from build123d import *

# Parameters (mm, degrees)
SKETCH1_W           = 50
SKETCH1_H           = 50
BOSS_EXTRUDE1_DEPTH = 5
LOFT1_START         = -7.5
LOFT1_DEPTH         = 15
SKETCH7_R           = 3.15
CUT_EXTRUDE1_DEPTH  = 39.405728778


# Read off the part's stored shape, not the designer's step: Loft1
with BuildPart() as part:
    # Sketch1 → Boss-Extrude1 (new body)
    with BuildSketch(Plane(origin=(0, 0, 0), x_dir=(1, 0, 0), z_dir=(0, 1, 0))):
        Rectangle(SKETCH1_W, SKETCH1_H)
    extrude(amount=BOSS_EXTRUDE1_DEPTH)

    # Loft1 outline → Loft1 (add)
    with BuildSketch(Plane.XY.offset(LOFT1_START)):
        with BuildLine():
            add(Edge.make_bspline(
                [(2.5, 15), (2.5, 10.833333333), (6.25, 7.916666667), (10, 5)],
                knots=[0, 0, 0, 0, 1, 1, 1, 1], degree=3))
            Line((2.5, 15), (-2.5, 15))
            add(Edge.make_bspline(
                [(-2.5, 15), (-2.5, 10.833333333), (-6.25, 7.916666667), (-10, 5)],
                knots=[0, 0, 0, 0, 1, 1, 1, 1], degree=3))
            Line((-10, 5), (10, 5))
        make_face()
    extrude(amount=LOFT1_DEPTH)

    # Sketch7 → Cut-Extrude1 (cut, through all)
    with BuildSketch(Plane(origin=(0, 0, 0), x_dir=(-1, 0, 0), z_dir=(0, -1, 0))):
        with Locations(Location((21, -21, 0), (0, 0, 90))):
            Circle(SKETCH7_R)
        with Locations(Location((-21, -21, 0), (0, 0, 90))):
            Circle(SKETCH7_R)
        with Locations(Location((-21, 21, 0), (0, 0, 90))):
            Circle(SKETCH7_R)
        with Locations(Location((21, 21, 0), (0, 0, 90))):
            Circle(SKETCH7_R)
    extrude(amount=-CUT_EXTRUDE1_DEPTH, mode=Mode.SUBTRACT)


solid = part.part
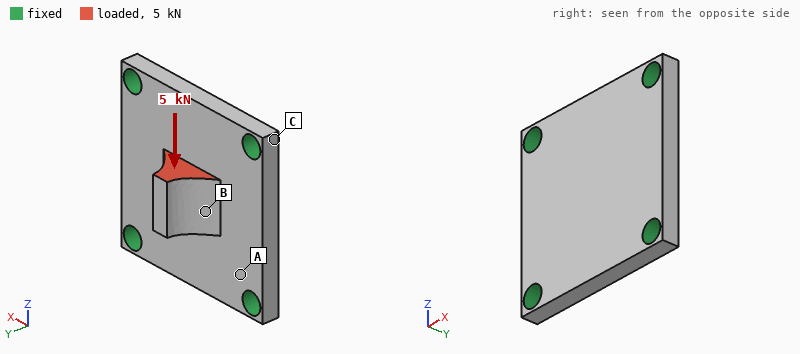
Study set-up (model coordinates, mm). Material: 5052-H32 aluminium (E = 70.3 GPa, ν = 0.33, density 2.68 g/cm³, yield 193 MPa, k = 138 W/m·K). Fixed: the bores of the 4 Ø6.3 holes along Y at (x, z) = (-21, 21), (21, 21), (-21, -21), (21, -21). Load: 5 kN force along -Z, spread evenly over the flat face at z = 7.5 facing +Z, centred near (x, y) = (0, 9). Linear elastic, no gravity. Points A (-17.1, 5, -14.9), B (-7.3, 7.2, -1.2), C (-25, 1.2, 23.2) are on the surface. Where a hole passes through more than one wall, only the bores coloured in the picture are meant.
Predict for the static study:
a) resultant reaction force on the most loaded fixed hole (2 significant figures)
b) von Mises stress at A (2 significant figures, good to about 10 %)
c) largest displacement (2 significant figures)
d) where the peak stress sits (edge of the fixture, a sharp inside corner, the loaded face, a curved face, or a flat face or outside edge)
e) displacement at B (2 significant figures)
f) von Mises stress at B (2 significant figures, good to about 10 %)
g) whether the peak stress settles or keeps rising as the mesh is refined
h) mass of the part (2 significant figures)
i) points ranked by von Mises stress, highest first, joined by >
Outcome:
1.5 kN
28 MPa
50 µm
edge of the fixture
17 µm
48 MPa
keeps rising
36 g
B > A > C
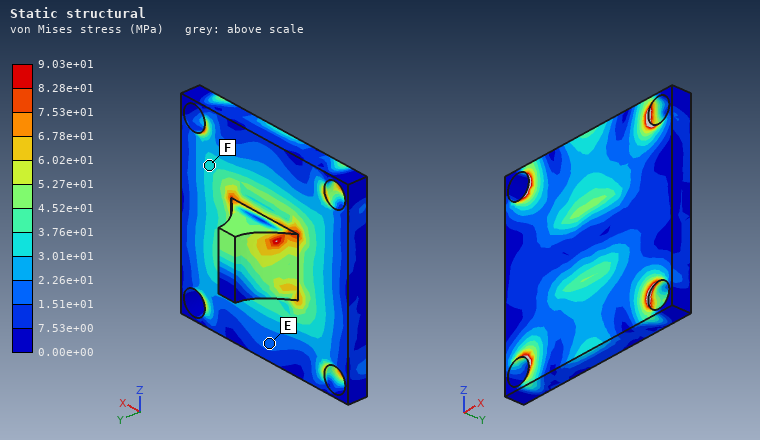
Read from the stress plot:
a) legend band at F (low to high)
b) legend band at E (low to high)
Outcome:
3.01e+01 to 3.76e+01 MPa
1.51e+01 to 2.26e+01 MPa
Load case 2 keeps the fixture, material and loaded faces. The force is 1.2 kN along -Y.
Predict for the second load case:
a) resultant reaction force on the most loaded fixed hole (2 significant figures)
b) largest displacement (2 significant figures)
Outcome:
440 N
29 µm
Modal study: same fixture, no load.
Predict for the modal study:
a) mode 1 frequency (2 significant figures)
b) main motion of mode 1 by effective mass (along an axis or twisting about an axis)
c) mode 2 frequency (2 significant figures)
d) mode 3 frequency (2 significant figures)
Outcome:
10 kHz
along Y
17 kHz
17 kHz
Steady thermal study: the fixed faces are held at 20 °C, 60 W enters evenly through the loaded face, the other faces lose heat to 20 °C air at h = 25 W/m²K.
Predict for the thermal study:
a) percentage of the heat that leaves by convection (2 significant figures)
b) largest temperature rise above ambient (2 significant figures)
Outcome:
3.1 %
55 K
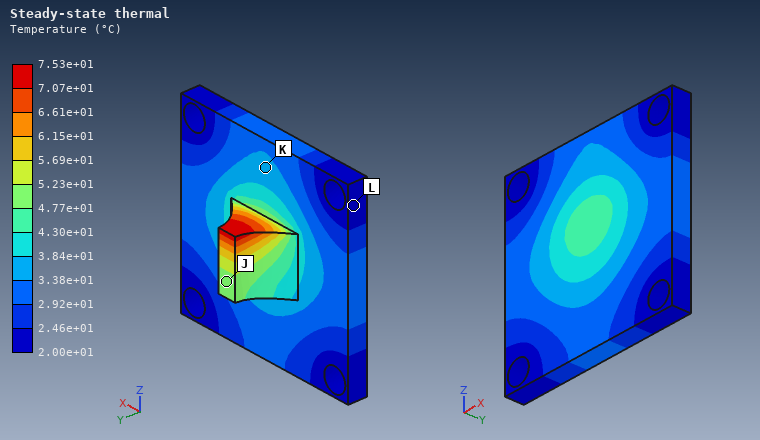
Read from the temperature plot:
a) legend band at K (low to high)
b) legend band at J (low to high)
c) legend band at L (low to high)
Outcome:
3.38e+01 to 3.84e+01 °C
4.77e+01 to 5.23e+01 °C
2.00e+01 to 2.46e+01 °C
